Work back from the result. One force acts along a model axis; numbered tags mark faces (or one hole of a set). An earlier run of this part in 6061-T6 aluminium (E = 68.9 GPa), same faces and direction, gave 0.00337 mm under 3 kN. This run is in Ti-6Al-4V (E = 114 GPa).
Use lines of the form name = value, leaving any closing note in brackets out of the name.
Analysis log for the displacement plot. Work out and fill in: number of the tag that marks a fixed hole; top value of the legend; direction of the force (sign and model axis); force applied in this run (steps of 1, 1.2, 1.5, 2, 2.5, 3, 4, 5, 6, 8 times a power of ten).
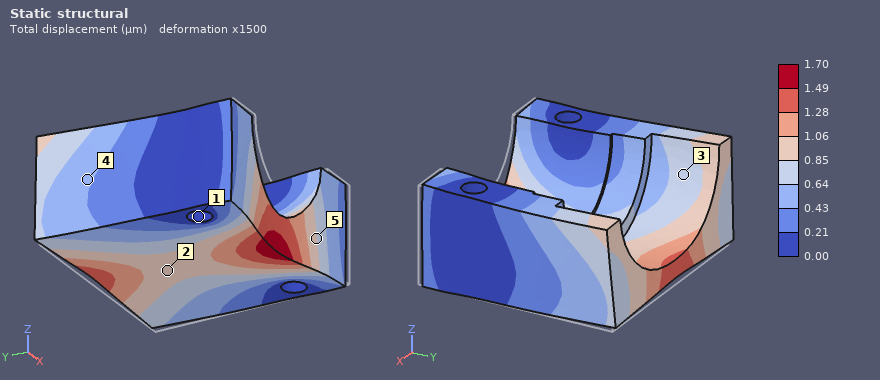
number of the tag that marks a fixed hole = 1
top value of the legend = 1.70 µm
direction of the force = +Y
force applied in this run = 2.5 kN
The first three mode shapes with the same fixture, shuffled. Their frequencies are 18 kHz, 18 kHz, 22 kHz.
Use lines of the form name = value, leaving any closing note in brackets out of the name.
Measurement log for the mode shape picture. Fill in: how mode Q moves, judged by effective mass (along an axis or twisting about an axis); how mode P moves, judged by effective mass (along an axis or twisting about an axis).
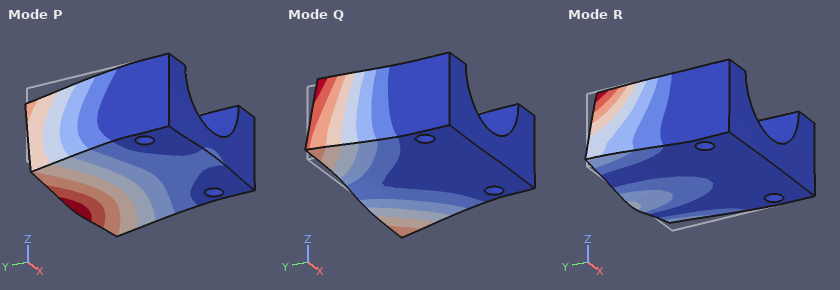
how mode Q moves, judged by effective mass = along X
how mode P moves, judged by effective mass = along Z
